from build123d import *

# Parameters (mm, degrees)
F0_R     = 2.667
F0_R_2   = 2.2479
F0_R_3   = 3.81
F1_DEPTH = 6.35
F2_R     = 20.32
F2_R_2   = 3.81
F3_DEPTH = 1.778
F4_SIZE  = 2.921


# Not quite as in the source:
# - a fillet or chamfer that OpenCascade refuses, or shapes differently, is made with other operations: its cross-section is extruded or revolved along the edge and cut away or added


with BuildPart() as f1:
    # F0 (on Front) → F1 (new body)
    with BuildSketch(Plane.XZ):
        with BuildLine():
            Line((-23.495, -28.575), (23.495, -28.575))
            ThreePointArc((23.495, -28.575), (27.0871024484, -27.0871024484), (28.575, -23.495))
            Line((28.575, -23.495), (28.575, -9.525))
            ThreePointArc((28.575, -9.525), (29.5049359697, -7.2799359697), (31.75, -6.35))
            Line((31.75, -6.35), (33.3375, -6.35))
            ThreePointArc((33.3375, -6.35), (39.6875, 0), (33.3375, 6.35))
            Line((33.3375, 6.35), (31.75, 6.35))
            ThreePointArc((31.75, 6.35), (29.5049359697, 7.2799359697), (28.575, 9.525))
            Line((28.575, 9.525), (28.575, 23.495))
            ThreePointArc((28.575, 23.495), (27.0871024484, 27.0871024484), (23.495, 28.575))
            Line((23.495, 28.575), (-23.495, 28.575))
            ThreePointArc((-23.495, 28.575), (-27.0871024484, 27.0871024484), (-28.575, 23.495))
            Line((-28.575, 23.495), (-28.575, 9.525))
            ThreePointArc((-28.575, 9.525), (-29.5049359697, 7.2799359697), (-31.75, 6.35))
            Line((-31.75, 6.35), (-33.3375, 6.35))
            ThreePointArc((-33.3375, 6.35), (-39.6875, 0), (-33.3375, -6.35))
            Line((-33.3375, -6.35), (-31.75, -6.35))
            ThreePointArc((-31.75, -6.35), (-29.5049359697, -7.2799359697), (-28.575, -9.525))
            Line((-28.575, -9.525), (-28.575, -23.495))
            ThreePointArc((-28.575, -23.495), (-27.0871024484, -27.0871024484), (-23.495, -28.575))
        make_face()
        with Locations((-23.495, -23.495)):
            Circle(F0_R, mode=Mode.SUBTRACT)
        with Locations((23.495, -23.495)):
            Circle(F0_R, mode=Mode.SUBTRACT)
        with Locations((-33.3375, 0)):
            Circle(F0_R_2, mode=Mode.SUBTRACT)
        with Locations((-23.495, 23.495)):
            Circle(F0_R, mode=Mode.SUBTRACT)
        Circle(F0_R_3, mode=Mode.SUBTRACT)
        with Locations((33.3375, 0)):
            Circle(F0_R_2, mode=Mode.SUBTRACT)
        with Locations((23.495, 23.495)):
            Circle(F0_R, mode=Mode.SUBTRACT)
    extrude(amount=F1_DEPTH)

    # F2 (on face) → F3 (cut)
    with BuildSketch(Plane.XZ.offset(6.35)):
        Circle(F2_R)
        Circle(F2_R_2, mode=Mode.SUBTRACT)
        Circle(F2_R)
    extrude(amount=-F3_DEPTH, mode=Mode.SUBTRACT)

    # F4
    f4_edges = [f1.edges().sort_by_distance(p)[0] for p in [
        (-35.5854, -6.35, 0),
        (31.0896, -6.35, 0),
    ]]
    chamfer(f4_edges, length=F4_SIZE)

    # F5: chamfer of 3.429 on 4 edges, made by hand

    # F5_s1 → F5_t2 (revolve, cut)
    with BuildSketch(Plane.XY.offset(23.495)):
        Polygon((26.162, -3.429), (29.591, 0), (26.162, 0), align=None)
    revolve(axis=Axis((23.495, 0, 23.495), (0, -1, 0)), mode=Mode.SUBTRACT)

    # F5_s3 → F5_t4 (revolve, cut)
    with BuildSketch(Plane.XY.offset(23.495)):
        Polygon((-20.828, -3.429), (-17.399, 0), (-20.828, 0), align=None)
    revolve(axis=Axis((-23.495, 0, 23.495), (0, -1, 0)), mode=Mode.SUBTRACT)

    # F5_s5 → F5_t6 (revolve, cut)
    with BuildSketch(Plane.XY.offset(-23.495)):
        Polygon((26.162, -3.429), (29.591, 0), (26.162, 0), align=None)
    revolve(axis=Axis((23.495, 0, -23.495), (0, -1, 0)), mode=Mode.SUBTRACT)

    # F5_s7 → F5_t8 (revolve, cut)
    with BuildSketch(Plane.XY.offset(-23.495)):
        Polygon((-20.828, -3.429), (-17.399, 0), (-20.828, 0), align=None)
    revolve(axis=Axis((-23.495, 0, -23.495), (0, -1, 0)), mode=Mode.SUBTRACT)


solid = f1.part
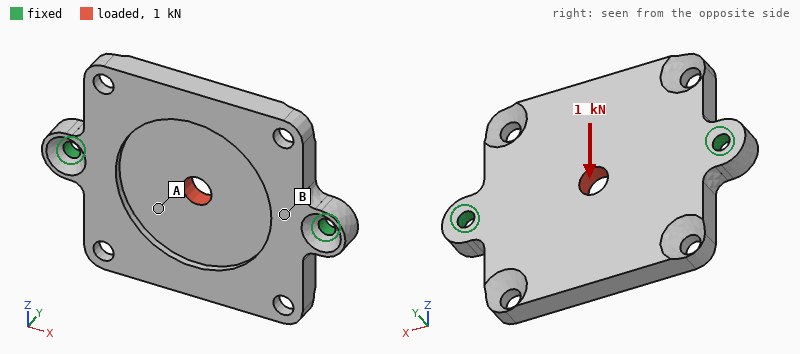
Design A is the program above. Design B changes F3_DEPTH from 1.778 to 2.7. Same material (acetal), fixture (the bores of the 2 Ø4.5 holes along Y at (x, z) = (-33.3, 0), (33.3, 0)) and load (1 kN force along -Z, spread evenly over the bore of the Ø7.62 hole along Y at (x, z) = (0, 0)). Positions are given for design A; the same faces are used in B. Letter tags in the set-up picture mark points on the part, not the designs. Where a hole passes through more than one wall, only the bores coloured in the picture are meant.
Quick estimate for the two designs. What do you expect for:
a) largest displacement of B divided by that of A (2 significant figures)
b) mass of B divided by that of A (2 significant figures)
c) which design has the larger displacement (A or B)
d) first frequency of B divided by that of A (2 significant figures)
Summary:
1.6
0.94
B
0.99
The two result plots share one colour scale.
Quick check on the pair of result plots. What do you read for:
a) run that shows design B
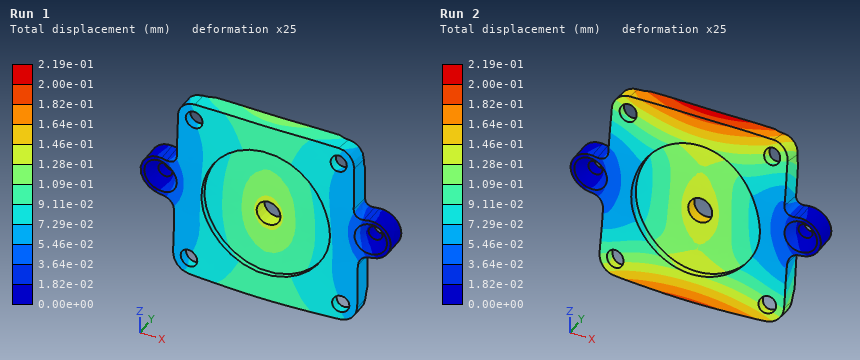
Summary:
Run 2
